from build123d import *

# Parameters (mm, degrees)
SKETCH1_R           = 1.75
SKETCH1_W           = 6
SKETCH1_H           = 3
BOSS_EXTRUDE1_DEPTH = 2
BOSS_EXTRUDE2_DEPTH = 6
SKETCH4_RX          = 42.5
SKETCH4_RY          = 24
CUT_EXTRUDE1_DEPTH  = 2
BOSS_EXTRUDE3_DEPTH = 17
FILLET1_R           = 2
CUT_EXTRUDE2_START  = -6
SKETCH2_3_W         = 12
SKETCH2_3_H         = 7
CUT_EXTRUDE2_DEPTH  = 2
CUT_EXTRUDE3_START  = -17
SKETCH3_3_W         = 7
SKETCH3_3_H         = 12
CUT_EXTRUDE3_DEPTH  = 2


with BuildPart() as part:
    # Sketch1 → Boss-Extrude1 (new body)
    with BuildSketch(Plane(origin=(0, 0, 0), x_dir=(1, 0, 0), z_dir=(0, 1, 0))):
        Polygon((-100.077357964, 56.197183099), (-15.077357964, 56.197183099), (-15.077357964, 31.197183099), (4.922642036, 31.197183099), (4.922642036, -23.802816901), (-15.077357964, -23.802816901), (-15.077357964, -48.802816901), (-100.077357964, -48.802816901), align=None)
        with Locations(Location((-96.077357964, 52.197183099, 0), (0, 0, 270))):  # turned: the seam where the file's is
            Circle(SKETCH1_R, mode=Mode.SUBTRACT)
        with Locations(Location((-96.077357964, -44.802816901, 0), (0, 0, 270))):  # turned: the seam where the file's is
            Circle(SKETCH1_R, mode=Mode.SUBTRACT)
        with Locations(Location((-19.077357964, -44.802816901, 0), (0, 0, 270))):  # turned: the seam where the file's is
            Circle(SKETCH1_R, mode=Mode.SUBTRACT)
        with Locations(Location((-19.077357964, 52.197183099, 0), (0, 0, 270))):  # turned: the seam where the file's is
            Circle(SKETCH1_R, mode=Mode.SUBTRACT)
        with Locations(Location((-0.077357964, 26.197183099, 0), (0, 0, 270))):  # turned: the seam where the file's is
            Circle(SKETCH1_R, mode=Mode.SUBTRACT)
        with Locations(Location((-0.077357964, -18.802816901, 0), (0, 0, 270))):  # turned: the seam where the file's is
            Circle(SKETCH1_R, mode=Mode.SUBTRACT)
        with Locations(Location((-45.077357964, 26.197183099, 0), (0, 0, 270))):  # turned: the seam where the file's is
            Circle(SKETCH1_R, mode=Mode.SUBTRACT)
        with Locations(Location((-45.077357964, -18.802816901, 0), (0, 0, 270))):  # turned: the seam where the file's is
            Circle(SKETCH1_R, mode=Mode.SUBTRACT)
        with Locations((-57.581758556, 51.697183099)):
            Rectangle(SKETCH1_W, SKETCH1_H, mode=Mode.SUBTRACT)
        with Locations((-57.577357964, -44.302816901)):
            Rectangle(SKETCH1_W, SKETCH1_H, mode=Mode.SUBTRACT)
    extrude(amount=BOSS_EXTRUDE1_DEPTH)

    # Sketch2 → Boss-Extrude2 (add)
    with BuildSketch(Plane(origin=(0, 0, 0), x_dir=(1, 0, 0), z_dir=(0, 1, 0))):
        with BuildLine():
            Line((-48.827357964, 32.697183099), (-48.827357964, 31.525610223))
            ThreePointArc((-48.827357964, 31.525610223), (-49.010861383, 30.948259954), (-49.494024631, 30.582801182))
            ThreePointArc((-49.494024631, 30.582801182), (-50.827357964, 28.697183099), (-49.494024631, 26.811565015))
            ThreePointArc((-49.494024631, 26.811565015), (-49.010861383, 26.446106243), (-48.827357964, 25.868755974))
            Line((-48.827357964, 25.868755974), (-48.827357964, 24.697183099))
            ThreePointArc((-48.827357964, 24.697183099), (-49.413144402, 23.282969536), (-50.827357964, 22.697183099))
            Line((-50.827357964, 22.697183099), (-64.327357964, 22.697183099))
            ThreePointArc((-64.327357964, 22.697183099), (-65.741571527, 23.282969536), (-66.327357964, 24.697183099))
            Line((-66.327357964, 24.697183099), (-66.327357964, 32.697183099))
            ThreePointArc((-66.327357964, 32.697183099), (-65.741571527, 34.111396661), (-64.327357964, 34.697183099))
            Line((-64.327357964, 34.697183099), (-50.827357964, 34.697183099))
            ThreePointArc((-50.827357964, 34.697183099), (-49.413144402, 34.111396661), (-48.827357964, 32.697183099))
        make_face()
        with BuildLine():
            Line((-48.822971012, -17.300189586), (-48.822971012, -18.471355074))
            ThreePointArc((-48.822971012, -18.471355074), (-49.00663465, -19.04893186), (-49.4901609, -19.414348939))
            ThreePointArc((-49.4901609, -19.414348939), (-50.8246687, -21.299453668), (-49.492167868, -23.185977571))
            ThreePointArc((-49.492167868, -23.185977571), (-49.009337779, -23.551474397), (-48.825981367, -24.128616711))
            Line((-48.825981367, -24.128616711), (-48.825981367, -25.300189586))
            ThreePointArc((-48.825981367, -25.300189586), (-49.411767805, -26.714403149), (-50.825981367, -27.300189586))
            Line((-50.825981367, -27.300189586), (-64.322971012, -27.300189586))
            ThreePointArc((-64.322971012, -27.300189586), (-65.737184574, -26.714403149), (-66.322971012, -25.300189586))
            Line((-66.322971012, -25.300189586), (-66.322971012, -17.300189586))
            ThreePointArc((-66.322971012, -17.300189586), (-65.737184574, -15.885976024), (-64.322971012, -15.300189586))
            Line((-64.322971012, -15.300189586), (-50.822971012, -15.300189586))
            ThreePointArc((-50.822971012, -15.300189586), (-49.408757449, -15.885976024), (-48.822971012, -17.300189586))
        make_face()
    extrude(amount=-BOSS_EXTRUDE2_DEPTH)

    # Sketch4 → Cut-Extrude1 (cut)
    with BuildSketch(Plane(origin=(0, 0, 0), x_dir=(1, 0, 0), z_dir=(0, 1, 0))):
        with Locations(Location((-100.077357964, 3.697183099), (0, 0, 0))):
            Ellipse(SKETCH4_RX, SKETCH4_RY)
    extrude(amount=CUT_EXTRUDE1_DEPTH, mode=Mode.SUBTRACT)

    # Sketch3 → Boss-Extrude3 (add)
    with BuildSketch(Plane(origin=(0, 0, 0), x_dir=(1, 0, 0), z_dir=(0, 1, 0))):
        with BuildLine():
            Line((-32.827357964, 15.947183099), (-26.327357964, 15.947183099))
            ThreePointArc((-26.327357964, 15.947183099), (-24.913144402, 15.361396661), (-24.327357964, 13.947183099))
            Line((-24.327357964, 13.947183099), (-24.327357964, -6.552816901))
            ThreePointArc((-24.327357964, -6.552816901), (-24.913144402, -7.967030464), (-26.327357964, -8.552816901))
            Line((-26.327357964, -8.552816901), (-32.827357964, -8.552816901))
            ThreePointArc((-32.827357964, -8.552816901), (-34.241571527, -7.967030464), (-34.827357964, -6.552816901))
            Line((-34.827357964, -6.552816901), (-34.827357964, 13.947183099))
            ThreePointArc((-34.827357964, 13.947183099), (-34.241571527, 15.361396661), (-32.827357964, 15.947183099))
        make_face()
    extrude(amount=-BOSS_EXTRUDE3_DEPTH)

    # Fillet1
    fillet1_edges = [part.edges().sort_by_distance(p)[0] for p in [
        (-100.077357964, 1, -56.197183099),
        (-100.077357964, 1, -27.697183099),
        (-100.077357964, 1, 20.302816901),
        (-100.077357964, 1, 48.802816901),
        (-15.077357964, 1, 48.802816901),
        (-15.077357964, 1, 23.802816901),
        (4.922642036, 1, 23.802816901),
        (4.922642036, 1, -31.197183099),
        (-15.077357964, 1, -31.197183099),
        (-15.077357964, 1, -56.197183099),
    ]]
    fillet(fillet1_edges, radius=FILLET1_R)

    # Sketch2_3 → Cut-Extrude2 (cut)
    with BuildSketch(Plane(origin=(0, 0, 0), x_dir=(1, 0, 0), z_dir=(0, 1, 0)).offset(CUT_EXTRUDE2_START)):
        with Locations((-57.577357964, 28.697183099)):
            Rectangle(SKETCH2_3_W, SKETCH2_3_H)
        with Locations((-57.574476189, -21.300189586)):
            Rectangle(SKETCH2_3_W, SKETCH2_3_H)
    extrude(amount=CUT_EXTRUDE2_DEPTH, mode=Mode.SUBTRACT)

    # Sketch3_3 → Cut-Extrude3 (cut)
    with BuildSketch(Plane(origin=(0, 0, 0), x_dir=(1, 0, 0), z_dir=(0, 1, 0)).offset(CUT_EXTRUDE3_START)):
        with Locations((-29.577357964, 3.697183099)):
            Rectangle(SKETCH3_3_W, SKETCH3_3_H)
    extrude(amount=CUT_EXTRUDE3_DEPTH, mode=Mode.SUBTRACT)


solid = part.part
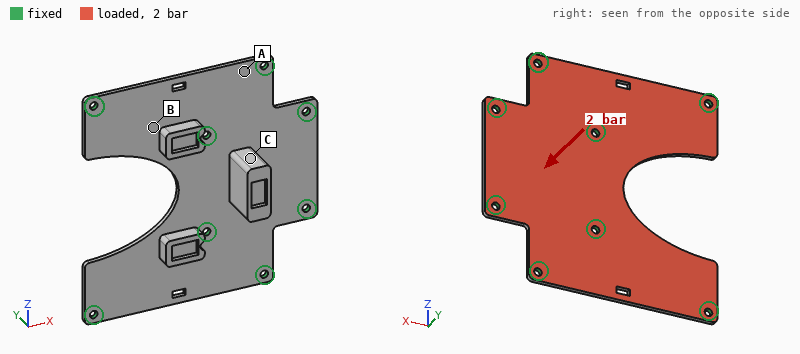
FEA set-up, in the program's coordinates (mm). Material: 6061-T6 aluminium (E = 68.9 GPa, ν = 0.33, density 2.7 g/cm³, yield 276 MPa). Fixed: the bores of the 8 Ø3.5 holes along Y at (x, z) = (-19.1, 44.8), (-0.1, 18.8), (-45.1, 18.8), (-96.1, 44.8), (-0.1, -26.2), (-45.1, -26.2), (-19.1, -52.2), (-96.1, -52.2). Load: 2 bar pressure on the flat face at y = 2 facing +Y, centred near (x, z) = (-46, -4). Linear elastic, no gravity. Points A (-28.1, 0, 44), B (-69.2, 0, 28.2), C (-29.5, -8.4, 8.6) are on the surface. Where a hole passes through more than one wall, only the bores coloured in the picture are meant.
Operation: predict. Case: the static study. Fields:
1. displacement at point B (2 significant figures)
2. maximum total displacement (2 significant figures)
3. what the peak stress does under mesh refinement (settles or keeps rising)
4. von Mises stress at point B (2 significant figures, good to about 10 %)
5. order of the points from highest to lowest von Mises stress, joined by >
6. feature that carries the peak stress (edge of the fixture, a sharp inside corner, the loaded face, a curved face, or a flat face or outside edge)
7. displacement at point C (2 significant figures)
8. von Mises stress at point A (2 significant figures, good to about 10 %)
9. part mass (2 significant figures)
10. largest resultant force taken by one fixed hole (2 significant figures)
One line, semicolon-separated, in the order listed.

0.14 mm; 0.19 mm; keeps rising; 44 MPa; B > A > C; edge of the fixture; 0.052 mm; 23 MPa; 62 g; 420 N
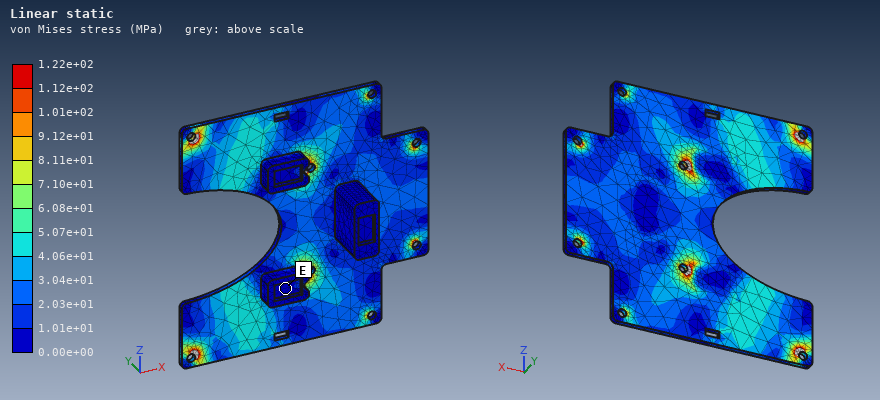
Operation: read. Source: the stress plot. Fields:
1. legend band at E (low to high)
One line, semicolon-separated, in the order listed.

0.00e+00 to 1.01e+01 MPa
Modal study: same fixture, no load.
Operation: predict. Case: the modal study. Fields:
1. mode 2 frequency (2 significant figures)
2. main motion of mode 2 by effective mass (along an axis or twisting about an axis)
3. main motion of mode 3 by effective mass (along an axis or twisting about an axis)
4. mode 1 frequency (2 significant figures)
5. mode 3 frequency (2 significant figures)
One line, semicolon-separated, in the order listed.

2600 Hz; twisting about X; along Y; 2500 Hz; 2700 Hz
